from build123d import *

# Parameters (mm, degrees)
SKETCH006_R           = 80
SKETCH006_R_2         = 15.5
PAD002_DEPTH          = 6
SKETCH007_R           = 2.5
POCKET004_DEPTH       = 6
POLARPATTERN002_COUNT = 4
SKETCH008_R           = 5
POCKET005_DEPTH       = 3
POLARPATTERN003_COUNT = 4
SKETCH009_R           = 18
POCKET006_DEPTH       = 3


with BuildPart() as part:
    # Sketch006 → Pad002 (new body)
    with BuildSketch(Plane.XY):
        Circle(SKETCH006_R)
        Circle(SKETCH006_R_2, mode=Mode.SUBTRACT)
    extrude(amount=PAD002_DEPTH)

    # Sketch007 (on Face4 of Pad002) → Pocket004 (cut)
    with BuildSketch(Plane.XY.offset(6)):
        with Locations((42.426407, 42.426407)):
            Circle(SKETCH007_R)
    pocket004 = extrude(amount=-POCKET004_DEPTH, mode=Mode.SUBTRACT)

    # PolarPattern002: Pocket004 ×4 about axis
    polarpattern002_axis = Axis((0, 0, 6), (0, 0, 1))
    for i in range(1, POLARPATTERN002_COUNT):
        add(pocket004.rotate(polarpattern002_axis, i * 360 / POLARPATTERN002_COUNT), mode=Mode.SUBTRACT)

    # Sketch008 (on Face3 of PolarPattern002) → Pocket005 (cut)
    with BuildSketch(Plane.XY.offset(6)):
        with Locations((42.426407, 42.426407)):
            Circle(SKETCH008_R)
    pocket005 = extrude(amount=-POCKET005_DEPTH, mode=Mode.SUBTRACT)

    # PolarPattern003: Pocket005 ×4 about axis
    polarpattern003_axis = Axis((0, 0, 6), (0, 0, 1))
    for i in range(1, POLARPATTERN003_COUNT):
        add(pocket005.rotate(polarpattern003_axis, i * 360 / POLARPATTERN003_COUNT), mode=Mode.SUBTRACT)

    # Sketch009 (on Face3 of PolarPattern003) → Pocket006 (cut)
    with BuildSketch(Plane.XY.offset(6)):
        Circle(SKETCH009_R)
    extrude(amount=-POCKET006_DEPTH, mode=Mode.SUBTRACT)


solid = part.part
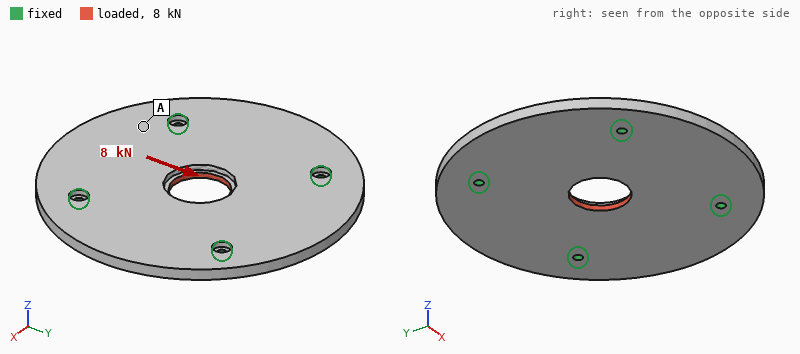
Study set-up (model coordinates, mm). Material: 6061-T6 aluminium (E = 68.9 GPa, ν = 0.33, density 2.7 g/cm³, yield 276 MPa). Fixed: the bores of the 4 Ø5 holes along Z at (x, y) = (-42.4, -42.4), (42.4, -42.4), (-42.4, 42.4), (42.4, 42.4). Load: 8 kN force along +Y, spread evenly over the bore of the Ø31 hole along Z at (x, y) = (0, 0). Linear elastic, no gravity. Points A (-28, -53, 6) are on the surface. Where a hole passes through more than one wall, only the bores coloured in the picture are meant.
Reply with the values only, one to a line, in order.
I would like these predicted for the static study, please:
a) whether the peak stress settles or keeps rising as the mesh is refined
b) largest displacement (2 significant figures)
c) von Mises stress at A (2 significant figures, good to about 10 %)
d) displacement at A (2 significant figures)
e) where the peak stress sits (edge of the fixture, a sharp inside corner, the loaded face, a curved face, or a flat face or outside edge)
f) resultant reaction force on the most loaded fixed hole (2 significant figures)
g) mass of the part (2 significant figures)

keeps rising
16 µm
6.8 MPa
7.3 µm
edge of the fixture
2.0 kN
310 g
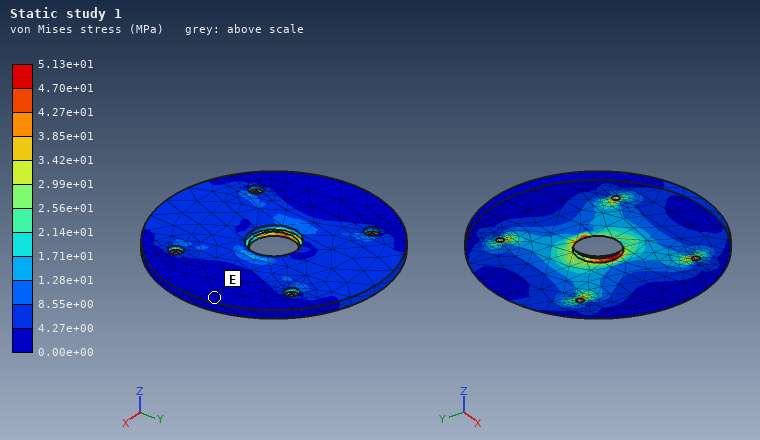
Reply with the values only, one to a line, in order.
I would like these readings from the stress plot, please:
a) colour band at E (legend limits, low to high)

0.00e+00 to 4.27e+00 MPa
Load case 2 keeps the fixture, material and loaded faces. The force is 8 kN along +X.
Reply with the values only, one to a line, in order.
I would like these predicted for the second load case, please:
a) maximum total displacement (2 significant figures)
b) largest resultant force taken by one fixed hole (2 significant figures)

16 µm
2.0 kN
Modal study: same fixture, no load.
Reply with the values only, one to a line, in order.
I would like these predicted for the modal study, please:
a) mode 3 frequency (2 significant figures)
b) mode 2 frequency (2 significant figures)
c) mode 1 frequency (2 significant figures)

2300 Hz
2300 Hz
1800 Hz
